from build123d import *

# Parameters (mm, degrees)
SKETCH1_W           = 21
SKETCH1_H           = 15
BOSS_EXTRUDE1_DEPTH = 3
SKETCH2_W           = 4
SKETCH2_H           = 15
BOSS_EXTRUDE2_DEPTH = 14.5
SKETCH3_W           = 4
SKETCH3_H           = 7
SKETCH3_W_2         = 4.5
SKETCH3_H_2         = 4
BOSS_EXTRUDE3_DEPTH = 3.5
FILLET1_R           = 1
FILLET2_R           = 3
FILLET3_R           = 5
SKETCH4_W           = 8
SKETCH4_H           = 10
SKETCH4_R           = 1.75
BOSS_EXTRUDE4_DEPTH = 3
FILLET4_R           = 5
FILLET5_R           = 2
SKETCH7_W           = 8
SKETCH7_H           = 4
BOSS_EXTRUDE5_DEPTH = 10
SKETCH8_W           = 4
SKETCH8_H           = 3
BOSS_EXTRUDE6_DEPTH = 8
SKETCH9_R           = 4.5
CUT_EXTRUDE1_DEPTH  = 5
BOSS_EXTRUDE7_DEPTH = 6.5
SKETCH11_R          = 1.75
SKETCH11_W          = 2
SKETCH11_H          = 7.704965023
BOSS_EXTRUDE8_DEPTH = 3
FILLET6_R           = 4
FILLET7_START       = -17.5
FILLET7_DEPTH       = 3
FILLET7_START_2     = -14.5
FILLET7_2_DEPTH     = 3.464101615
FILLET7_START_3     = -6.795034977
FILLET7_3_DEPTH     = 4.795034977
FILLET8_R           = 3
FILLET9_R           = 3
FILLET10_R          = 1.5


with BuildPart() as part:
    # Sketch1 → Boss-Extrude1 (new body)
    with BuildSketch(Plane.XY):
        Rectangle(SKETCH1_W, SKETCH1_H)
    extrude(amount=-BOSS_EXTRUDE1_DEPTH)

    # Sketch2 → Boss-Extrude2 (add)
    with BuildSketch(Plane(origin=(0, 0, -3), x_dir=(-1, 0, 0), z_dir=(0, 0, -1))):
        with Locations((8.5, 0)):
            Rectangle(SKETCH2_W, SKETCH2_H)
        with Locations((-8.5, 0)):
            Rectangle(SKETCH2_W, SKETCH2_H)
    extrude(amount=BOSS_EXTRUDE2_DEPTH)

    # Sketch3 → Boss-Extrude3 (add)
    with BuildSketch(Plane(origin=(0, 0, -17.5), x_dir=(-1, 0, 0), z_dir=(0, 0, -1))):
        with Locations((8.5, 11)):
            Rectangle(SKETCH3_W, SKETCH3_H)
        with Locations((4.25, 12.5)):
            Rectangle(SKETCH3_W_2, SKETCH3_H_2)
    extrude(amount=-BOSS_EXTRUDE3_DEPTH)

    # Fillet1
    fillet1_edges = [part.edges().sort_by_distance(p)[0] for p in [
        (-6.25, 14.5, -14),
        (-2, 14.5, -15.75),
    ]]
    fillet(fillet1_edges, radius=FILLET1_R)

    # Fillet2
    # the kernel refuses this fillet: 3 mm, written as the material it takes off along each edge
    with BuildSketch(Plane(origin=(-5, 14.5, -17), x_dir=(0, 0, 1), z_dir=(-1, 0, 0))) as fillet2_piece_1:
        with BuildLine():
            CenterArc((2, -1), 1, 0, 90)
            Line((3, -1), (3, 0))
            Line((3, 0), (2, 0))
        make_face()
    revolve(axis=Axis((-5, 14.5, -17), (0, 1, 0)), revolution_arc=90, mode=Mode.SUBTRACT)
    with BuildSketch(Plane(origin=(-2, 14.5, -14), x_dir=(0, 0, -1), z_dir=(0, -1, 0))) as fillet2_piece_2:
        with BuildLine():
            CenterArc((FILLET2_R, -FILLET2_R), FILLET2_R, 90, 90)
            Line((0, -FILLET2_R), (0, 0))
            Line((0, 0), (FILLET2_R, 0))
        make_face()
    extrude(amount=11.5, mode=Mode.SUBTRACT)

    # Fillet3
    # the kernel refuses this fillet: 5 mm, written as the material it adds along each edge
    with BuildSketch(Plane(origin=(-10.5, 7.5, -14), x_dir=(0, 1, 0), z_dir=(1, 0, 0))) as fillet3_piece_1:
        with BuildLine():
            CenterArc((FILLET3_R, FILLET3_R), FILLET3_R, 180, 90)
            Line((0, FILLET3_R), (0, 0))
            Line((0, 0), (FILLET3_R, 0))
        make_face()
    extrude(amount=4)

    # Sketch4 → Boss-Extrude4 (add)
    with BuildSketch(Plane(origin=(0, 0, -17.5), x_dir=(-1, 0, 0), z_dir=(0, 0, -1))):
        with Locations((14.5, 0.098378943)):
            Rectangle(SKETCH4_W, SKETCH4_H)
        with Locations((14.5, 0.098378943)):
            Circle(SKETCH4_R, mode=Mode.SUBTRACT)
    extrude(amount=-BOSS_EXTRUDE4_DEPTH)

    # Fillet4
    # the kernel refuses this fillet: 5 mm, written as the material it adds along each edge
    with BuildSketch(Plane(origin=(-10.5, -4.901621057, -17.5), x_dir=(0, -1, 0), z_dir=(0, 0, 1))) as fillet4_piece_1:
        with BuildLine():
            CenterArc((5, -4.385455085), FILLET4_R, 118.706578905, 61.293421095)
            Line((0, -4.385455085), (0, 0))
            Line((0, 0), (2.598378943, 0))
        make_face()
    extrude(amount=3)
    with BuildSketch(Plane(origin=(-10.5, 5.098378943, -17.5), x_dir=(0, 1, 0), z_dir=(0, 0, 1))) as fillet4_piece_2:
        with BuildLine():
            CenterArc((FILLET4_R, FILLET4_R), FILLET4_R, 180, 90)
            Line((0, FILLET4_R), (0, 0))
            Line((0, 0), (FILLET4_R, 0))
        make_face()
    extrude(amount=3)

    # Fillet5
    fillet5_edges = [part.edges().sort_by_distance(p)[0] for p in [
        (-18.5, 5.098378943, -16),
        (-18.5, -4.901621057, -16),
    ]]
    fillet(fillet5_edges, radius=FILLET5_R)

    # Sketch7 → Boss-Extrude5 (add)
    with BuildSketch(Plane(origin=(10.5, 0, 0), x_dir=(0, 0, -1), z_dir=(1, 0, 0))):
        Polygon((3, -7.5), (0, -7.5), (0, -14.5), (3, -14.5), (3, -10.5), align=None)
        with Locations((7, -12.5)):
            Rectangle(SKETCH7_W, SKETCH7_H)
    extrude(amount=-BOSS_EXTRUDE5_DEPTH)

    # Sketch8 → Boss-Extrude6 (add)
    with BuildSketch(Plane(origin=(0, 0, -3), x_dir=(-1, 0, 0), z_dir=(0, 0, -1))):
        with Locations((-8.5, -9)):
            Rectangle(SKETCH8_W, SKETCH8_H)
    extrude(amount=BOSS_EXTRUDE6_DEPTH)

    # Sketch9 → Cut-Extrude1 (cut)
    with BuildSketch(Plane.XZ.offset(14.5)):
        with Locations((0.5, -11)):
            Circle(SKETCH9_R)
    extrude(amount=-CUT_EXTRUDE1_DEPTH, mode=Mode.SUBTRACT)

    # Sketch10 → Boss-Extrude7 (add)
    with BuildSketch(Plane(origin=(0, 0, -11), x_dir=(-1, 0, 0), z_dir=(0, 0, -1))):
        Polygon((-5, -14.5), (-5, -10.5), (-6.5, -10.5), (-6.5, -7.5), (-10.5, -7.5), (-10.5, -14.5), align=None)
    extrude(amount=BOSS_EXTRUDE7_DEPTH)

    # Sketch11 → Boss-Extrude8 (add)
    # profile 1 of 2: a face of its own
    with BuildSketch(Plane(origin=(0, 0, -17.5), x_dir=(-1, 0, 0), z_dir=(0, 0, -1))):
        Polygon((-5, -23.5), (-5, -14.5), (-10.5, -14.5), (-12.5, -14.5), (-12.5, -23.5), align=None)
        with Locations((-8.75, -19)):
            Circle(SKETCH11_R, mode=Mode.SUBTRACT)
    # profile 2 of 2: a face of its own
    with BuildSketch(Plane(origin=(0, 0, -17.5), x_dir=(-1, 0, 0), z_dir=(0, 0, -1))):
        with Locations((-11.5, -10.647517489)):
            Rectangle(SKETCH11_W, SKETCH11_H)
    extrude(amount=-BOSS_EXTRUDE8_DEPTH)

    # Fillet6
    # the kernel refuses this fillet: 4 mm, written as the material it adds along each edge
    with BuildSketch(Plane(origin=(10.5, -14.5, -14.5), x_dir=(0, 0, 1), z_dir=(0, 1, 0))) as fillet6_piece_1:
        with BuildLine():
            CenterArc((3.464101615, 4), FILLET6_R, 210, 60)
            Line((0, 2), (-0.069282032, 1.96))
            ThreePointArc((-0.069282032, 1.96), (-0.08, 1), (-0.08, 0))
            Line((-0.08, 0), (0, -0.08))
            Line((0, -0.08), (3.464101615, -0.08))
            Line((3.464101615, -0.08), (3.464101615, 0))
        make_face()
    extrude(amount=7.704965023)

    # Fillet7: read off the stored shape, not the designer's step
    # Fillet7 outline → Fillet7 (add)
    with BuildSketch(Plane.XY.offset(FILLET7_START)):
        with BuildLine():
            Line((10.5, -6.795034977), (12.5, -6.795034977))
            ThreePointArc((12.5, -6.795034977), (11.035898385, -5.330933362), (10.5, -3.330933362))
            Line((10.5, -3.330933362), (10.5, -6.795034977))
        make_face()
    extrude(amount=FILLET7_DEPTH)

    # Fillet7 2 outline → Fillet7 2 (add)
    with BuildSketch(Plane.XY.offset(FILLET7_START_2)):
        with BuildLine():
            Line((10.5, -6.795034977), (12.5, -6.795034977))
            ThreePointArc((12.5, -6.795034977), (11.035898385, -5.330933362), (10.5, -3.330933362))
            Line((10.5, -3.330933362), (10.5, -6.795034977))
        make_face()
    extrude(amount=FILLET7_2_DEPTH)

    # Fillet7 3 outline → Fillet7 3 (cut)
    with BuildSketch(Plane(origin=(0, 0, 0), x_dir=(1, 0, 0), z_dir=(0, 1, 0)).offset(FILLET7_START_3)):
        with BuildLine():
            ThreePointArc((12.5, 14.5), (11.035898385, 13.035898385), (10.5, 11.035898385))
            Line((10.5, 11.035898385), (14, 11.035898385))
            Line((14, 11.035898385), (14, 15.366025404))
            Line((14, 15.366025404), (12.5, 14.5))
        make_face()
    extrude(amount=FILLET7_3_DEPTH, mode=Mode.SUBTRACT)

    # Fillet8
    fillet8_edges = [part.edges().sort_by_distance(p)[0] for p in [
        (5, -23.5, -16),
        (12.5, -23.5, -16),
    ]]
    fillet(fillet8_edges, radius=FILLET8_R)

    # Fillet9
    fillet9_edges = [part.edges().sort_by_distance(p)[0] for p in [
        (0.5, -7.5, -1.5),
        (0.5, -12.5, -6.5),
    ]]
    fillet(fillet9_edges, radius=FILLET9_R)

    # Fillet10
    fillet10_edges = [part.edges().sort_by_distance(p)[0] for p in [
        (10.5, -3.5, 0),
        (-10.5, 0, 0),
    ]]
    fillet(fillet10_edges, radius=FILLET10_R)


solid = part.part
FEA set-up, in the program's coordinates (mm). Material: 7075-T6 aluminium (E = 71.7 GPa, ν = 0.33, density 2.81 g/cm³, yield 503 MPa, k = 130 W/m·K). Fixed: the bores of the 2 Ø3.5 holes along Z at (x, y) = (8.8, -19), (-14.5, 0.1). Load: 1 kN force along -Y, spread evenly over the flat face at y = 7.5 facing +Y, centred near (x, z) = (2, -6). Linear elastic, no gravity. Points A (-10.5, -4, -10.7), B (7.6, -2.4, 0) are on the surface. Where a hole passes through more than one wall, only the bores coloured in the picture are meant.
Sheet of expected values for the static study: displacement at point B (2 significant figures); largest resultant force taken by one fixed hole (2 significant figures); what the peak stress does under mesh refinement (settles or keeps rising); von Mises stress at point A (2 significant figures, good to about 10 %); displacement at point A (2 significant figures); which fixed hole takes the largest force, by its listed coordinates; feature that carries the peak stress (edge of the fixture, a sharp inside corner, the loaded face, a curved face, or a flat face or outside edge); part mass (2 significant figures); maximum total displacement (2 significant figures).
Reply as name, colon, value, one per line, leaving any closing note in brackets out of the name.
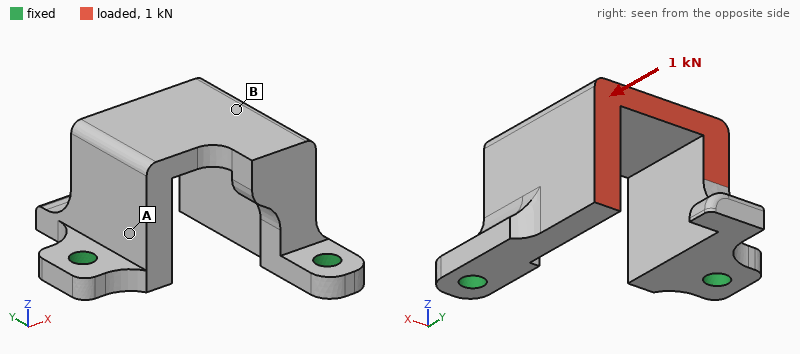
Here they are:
displacement at point B: 0.19 mm
largest resultant force taken by one fixed hole: 580 N
what the peak stress does under mesh refinement: keeps rising
von Mises stress at point A: 62 MPa
displacement at point A: 0.056 mm
which fixed hole takes the largest force, by its listed coordinates: (8.8, -19)
feature that carries the peak stress: edge of the fixture
part mass: 11 g
maximum total displacement: 0.25 mm
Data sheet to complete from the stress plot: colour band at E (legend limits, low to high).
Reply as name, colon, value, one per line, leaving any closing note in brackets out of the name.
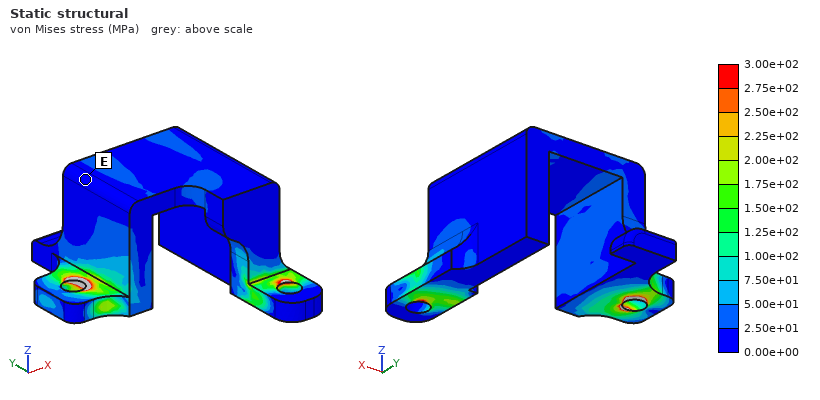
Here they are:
colour band at E: 0.00e+00 to 2.50e+01 MPa
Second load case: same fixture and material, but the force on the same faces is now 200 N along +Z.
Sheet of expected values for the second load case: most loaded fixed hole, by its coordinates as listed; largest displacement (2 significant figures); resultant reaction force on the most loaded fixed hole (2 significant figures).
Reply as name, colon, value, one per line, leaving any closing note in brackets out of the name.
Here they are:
most loaded fixed hole, by its coordinates as listed: (-14.5, 0.1)
largest displacement: 97 µm
resultant reaction force on the most loaded fixed hole: 150 N
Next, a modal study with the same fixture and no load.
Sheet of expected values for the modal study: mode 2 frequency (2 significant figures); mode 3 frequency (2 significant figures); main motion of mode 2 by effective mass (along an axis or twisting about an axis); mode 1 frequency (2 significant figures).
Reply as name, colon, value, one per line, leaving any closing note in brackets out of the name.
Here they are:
mode 2 frequency: 6800 Hz
mode 3 frequency: 10 kHz
main motion of mode 2 by effective mass: along X
mode 1 frequency: 3400 Hz
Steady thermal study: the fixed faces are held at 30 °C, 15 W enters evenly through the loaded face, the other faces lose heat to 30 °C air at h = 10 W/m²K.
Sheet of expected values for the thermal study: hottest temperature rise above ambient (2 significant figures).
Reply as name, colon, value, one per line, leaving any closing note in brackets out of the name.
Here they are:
hottest temperature rise above ambient: 30 K
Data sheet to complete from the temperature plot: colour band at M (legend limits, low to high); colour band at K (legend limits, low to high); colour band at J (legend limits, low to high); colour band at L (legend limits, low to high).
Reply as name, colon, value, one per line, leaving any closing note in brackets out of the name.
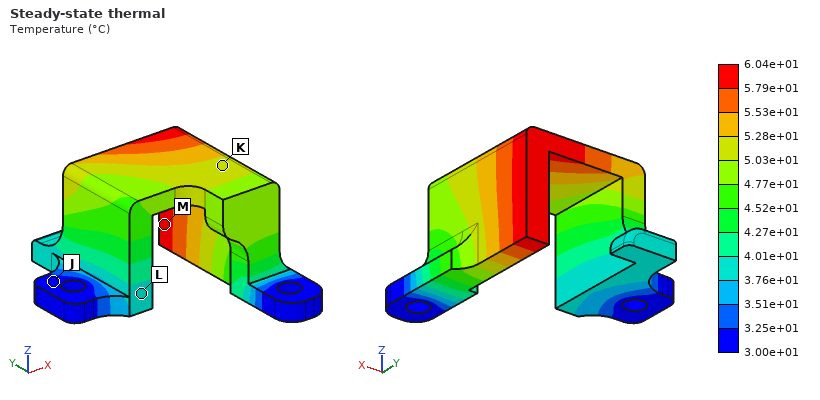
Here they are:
colour band at M: 5.79e+01 to 6.04e+01 °C
colour band at K: 5.03e+01 to 5.28e+01 °C
colour band at J: 3.00e+01 to 3.25e+01 °C
colour band at L: 3.76e+01 to 4.01e+01 °C
